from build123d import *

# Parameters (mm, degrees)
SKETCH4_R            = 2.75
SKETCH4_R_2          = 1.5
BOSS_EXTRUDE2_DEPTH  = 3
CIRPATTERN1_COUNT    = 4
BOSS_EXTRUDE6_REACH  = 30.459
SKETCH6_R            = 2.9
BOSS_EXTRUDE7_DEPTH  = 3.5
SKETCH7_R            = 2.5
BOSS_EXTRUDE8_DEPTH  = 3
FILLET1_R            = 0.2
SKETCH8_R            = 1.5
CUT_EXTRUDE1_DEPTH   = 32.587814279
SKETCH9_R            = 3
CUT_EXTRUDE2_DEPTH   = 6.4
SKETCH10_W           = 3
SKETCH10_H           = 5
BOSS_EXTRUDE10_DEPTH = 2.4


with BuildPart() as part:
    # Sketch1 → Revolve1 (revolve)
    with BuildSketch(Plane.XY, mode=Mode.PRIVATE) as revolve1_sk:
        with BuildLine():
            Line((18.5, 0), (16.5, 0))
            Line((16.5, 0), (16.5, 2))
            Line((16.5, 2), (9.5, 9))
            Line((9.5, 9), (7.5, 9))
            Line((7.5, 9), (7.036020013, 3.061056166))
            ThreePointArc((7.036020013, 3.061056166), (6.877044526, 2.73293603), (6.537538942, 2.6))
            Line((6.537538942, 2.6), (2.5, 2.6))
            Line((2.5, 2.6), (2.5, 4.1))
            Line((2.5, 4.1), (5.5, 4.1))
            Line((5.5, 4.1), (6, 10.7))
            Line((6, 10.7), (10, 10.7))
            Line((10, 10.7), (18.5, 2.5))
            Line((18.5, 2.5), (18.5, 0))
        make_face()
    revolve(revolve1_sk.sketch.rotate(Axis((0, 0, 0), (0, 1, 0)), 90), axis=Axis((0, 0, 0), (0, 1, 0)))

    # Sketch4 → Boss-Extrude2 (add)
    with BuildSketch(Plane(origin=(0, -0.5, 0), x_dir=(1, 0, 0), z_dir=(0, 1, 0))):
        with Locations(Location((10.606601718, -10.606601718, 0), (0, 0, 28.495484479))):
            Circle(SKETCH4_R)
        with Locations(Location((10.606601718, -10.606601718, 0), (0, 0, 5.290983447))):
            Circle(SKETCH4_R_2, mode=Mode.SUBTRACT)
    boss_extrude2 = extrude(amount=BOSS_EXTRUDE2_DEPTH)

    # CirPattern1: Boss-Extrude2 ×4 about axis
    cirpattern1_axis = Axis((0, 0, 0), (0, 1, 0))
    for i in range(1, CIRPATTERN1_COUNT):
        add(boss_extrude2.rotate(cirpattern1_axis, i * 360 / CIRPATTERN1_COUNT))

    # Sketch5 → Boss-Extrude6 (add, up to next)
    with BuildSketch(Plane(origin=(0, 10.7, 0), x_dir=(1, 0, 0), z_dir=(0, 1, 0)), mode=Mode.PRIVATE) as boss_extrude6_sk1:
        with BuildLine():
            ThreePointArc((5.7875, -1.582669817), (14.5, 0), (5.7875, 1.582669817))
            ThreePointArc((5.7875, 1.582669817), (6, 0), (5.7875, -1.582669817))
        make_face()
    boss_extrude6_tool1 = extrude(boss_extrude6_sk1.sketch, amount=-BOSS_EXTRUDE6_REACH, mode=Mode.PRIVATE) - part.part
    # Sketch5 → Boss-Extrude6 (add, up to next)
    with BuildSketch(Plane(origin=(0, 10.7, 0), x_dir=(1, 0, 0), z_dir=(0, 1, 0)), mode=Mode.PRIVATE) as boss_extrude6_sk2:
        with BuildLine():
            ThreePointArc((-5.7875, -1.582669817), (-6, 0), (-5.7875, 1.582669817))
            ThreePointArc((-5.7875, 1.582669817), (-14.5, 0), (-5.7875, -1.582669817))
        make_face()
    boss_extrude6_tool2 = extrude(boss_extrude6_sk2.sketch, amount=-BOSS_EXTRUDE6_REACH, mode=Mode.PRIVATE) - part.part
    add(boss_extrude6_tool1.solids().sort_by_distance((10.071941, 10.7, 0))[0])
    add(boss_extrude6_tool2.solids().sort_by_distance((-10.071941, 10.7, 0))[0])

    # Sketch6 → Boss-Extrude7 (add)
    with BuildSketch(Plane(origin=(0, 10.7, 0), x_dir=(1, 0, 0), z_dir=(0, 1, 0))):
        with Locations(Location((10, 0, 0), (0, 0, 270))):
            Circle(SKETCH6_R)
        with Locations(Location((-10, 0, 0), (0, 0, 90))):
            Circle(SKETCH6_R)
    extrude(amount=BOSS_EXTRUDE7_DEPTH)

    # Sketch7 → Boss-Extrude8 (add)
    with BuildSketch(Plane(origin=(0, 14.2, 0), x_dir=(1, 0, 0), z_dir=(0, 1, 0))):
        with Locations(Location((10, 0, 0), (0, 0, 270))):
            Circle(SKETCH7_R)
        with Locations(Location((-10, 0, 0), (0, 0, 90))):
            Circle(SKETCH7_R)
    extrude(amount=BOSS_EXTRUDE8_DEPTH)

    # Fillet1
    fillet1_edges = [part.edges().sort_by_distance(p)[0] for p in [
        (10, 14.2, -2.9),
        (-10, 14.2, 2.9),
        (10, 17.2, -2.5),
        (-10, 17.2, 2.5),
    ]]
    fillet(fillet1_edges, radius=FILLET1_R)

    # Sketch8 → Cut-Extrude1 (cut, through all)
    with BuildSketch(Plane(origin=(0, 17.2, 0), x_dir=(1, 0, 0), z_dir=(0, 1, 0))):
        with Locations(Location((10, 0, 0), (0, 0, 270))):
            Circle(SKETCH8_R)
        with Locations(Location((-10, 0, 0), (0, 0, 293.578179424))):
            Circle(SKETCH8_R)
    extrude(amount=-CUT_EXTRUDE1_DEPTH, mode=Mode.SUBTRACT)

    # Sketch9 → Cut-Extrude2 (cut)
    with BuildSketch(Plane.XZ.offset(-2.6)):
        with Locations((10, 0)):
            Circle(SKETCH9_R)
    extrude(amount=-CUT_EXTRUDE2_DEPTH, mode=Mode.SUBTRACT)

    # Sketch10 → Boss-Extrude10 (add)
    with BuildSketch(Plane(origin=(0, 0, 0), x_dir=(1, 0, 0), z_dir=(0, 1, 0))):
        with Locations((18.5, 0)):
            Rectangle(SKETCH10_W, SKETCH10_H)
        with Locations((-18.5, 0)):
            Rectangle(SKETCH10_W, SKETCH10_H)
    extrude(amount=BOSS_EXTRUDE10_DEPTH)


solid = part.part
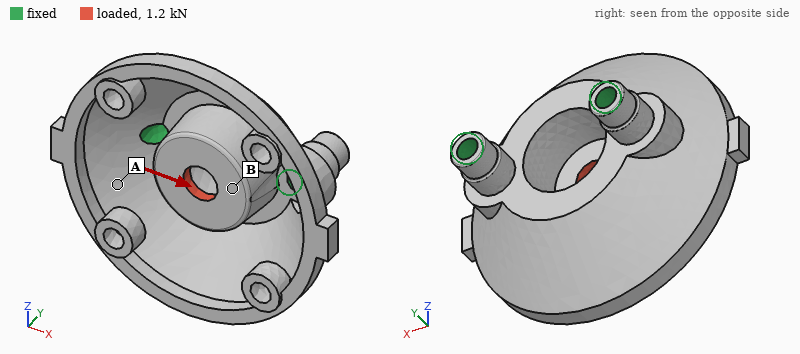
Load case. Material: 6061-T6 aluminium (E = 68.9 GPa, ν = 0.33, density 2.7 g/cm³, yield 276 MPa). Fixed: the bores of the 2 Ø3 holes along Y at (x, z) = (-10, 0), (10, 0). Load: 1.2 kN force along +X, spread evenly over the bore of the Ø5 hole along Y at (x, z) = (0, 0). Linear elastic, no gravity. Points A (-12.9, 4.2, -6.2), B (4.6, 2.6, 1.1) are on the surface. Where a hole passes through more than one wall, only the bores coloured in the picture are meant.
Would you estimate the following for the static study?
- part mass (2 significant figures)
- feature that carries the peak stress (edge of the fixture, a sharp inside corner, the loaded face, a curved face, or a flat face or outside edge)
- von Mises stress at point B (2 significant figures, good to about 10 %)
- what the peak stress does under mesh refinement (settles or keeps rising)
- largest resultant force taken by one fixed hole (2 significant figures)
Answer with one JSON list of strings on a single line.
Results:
["9.1 g", "a sharp inside corner", "64 MPa", "keeps rising", "790 N"]
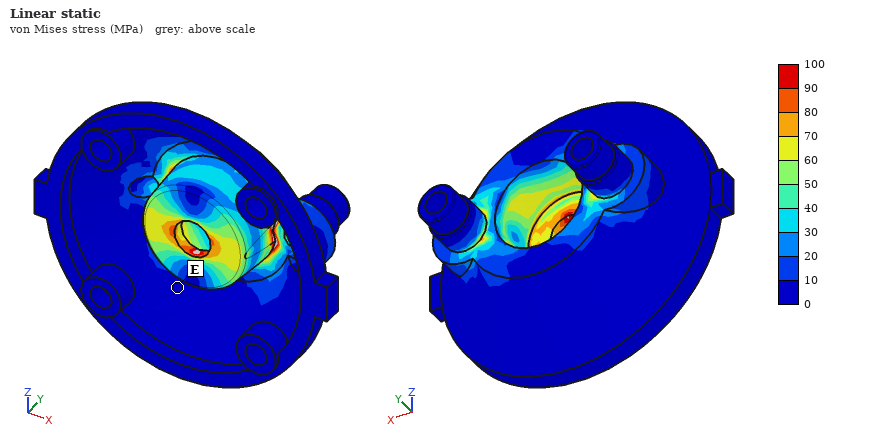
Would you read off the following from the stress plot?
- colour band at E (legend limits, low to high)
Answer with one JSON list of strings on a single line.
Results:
["0 to 10 MPa"]
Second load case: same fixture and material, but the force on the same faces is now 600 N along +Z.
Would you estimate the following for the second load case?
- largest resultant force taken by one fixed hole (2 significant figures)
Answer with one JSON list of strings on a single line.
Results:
["310 N"]
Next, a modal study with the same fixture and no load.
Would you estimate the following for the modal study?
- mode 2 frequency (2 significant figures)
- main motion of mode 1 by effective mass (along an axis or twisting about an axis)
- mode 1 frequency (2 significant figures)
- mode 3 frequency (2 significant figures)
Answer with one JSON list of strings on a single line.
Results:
["9300 Hz", "along Z", "7000 Hz", "9400 Hz"]
